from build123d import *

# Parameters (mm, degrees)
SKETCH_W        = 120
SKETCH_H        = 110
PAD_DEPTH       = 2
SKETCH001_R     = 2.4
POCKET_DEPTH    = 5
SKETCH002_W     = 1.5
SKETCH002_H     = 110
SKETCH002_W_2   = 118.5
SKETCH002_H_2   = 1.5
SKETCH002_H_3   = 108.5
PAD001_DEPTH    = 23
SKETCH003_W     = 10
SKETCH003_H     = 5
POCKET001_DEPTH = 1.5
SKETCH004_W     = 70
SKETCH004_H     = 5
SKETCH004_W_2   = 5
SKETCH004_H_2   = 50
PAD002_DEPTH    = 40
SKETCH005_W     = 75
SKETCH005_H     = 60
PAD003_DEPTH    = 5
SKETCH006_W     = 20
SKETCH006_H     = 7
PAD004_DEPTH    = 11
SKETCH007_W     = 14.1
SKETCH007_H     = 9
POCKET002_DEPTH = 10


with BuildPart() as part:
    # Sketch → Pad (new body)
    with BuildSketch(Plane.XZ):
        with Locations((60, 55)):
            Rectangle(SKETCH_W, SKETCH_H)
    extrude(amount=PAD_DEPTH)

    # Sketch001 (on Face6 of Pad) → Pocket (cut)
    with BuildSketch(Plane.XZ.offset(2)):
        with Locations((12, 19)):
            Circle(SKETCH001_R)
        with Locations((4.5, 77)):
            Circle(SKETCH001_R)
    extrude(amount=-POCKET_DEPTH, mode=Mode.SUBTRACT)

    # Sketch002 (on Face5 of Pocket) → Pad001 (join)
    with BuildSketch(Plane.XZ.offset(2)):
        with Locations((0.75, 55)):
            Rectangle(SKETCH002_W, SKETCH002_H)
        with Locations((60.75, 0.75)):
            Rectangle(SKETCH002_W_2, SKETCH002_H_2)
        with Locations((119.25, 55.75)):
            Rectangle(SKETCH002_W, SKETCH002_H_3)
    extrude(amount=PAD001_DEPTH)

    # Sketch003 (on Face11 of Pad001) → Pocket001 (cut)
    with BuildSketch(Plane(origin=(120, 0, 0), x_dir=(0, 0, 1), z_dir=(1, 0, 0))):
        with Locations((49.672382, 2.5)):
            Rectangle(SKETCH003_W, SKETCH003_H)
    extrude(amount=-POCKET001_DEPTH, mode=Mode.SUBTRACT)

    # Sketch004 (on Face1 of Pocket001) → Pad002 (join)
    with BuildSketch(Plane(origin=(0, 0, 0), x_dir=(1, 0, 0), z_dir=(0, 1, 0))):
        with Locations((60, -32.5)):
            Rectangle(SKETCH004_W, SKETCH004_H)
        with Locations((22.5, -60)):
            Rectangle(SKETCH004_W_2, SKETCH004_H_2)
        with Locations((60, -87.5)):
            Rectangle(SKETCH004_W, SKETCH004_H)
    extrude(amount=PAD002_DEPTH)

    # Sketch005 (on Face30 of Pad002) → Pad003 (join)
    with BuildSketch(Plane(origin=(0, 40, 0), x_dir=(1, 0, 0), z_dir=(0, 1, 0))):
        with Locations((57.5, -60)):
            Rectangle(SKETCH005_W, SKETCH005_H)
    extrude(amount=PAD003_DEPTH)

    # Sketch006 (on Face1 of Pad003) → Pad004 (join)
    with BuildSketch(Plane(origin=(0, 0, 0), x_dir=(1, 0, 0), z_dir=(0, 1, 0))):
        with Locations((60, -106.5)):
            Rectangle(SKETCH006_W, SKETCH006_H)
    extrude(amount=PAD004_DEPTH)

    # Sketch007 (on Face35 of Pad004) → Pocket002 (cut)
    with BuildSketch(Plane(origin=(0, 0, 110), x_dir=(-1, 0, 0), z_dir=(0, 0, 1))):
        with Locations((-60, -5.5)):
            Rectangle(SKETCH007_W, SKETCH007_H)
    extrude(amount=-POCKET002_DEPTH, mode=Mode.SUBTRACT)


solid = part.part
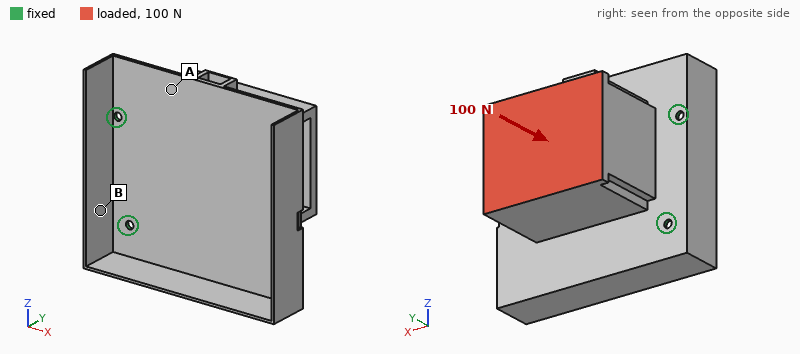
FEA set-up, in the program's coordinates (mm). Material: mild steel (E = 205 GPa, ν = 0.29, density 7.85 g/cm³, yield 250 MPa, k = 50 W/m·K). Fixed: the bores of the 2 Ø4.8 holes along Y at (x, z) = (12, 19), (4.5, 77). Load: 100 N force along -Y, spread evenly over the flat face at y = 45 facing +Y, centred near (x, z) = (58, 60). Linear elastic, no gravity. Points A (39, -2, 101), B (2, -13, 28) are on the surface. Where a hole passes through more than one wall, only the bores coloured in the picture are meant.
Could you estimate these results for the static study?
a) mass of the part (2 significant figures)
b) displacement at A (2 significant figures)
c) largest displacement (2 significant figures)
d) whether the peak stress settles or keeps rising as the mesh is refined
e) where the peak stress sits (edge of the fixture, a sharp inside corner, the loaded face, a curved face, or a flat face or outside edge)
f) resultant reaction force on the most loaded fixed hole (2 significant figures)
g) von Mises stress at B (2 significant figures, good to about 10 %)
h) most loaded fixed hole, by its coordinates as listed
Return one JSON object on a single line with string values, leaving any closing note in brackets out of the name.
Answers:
{"mass of the part": "780 g", "displacement at A": "0.11 mm", "largest displacement": "0.41 mm", "whether the peak stress settles or keeps rising as the mesh is refined": "keeps rising", "where the peak stress sits": "edge of the fixture", "resultant reaction force on the most loaded fixed hole": "65 N", "von Mises stress at B": "11 MPa", "most loaded fixed hole, by its coordinates as listed": "(4.5, 77)"}
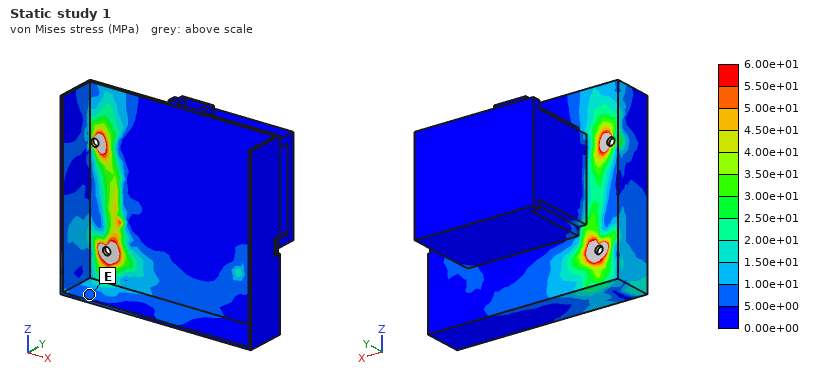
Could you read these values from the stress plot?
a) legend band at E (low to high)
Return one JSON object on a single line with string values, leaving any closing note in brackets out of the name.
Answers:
{"legend band at E": "5.00e+00 to 1.00e+01 MPa"}
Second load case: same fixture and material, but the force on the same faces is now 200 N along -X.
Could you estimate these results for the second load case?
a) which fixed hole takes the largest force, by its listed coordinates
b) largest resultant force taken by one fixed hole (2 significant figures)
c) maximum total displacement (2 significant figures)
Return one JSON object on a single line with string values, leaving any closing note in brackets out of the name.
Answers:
{"which fixed hole takes the largest force, by its listed coordinates": "(4.5, 77)", "largest resultant force taken by one fixed hole": "160 N", "maximum total displacement": "0.85 mm"}
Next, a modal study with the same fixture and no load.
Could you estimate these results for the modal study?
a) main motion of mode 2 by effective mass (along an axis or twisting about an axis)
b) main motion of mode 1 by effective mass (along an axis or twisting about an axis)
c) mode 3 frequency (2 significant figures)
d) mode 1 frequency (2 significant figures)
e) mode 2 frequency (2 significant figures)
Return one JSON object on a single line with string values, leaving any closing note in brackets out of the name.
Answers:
{"main motion of mode 2 by effective mass": "along Z", "main motion of mode 1 by effective mass": "along Y", "mode 3 frequency": "1000 Hz", "mode 1 frequency": "110 Hz", "mode 2 frequency": "540 Hz"}
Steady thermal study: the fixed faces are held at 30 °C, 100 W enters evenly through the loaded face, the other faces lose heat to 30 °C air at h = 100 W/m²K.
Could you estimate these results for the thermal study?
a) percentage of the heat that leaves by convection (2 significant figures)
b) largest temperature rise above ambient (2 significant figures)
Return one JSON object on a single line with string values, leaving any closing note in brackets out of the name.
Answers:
{"percentage of the heat that leaves by convection": "97 %", "largest temperature rise above ambient": "74 K"}
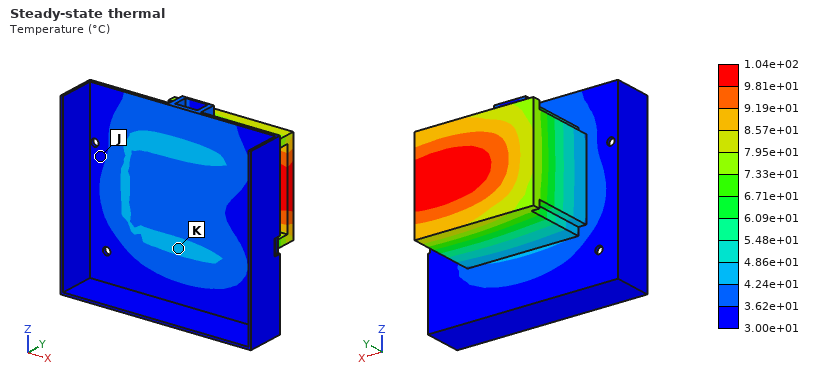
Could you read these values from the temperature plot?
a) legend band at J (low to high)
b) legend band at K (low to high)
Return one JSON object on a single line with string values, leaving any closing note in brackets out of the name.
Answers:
{"legend band at J": "3.00e+01 to 3.62e+01 °C", "legend band at K": "4.24e+01 to 4.86e+01 °C"}
